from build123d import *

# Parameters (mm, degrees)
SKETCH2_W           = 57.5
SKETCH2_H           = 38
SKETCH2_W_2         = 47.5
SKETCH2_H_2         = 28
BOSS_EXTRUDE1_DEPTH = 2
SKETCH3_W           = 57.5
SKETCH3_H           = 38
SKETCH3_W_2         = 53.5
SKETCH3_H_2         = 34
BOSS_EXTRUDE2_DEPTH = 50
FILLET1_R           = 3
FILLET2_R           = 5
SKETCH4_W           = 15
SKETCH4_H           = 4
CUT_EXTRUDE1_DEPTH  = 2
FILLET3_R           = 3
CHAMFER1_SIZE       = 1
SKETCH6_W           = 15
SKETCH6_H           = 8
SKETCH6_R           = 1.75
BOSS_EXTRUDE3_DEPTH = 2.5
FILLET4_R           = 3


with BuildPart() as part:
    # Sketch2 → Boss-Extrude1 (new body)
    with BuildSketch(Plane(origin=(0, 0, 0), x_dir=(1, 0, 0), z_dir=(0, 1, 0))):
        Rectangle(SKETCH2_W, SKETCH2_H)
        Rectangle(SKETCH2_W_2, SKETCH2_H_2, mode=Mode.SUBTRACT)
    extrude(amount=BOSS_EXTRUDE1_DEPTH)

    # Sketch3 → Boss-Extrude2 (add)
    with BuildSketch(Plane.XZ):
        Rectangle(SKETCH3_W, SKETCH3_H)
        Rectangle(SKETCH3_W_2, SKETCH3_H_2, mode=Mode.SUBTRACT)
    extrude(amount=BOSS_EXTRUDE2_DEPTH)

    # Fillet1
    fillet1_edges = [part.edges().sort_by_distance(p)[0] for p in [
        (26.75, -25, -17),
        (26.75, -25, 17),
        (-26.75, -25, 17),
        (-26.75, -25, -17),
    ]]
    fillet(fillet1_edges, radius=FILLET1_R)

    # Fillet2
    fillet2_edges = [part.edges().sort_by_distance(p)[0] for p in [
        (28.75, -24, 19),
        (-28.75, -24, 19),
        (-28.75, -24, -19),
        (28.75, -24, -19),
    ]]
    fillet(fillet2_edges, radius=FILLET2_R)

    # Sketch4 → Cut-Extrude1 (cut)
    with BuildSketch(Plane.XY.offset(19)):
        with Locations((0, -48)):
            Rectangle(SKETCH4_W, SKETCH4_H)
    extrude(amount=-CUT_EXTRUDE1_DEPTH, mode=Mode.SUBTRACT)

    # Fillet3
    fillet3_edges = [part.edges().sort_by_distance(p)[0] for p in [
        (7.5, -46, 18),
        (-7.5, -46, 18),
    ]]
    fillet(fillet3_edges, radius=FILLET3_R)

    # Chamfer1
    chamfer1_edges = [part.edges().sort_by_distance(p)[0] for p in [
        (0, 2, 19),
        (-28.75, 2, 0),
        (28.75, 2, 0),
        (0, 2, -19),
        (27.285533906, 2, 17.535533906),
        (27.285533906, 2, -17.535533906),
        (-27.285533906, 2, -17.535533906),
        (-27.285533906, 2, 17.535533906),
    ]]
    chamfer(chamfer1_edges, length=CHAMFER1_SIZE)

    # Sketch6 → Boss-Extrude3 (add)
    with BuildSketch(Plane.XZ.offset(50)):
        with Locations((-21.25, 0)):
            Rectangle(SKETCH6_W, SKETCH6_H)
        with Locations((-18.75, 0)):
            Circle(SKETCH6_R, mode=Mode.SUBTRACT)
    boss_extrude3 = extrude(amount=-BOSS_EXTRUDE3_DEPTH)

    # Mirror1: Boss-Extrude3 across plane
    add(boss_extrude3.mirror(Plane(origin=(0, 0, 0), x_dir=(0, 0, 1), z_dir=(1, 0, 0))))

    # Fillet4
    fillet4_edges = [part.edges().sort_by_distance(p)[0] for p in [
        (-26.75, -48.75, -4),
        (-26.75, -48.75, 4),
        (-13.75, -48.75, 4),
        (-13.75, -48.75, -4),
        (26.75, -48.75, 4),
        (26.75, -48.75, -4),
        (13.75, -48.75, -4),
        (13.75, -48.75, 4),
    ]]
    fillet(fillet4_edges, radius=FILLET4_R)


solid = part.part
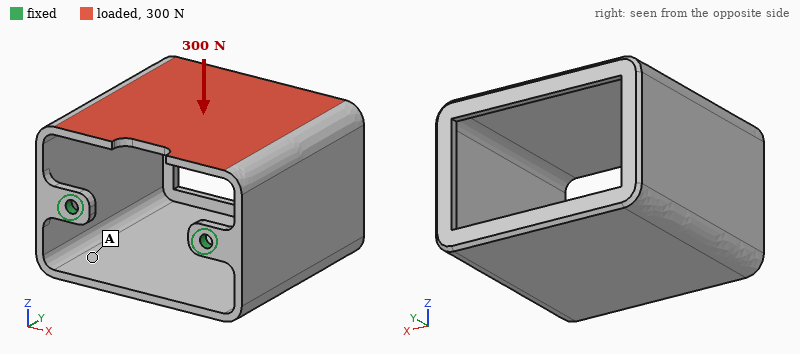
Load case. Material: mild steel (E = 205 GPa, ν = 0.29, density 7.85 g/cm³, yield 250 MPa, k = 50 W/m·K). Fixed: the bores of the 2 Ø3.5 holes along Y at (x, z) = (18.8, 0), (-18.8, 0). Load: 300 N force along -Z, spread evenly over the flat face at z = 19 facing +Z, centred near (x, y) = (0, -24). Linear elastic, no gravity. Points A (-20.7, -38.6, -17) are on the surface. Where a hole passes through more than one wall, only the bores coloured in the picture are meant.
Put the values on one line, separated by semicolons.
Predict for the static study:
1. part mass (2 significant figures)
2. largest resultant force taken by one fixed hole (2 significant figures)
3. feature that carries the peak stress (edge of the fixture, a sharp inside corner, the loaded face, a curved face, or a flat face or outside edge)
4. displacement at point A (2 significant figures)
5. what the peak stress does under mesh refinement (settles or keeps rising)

150 g; 160 N; edge of the fixture; 0.16 mm; keeps rising
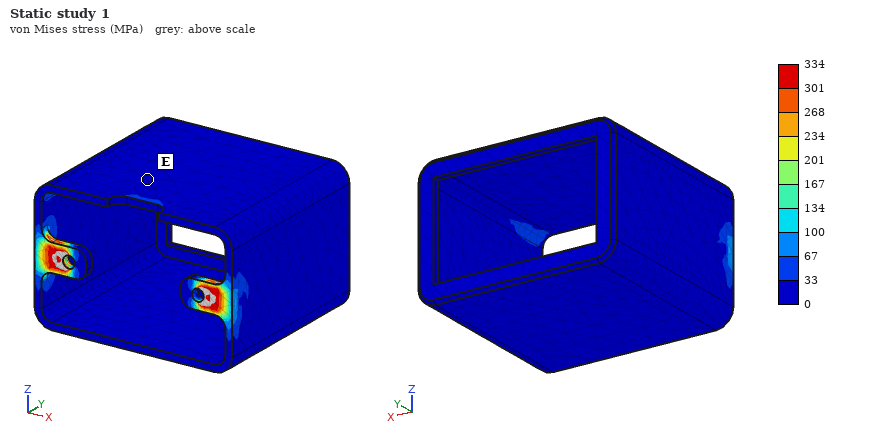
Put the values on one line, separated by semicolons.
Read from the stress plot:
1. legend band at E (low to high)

0 to 33 MPa
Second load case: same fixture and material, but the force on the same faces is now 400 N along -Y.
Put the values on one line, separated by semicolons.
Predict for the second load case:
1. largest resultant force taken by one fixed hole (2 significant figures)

200 N
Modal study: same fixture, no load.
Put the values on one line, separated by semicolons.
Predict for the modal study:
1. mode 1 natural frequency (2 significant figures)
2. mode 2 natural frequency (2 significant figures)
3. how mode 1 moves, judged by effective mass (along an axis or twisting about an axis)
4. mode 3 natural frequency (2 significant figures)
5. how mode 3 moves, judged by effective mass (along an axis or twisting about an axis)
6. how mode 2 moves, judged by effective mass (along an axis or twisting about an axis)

370 Hz; 1100 Hz; along Z; 1600 Hz; twisting about Y; along X
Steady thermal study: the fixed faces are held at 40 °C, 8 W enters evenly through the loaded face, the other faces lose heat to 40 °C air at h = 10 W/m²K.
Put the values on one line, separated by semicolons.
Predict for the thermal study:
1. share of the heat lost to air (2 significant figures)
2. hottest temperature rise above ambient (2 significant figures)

54 %; 41 K
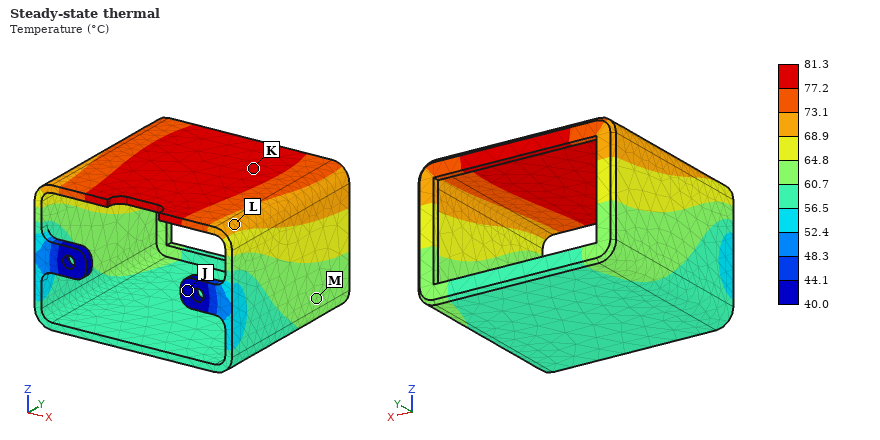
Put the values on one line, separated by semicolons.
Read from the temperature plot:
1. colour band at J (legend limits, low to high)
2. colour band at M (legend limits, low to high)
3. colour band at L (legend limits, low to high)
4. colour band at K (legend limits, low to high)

40.0 to 44.1 °C; 60.7 to 64.8 °C; 68.9 to 73.1 °C; 77.2 to 81.3 °C
